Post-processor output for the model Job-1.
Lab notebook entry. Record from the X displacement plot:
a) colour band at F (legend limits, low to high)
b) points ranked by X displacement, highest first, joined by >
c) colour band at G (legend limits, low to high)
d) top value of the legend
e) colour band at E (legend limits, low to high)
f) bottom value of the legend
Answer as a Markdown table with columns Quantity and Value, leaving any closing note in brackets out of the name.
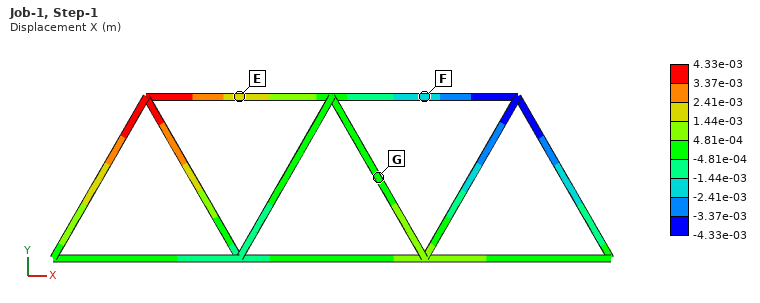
| Quantity | Value |
|---|---|
| colour band at F | -2.41e-03 to -1.44e-03 m |
| points ranked by X displacement, highest first, joined by > | E > G > F |
| colour band at G | -4.81e-04 to 4.81e-04 m |
| top value of the legend | 4.33e-03 m |
| colour band at E | 1.44e-03 to 2.41e-03 m |
| bottom value of the legend | -4.33e-03 m |
